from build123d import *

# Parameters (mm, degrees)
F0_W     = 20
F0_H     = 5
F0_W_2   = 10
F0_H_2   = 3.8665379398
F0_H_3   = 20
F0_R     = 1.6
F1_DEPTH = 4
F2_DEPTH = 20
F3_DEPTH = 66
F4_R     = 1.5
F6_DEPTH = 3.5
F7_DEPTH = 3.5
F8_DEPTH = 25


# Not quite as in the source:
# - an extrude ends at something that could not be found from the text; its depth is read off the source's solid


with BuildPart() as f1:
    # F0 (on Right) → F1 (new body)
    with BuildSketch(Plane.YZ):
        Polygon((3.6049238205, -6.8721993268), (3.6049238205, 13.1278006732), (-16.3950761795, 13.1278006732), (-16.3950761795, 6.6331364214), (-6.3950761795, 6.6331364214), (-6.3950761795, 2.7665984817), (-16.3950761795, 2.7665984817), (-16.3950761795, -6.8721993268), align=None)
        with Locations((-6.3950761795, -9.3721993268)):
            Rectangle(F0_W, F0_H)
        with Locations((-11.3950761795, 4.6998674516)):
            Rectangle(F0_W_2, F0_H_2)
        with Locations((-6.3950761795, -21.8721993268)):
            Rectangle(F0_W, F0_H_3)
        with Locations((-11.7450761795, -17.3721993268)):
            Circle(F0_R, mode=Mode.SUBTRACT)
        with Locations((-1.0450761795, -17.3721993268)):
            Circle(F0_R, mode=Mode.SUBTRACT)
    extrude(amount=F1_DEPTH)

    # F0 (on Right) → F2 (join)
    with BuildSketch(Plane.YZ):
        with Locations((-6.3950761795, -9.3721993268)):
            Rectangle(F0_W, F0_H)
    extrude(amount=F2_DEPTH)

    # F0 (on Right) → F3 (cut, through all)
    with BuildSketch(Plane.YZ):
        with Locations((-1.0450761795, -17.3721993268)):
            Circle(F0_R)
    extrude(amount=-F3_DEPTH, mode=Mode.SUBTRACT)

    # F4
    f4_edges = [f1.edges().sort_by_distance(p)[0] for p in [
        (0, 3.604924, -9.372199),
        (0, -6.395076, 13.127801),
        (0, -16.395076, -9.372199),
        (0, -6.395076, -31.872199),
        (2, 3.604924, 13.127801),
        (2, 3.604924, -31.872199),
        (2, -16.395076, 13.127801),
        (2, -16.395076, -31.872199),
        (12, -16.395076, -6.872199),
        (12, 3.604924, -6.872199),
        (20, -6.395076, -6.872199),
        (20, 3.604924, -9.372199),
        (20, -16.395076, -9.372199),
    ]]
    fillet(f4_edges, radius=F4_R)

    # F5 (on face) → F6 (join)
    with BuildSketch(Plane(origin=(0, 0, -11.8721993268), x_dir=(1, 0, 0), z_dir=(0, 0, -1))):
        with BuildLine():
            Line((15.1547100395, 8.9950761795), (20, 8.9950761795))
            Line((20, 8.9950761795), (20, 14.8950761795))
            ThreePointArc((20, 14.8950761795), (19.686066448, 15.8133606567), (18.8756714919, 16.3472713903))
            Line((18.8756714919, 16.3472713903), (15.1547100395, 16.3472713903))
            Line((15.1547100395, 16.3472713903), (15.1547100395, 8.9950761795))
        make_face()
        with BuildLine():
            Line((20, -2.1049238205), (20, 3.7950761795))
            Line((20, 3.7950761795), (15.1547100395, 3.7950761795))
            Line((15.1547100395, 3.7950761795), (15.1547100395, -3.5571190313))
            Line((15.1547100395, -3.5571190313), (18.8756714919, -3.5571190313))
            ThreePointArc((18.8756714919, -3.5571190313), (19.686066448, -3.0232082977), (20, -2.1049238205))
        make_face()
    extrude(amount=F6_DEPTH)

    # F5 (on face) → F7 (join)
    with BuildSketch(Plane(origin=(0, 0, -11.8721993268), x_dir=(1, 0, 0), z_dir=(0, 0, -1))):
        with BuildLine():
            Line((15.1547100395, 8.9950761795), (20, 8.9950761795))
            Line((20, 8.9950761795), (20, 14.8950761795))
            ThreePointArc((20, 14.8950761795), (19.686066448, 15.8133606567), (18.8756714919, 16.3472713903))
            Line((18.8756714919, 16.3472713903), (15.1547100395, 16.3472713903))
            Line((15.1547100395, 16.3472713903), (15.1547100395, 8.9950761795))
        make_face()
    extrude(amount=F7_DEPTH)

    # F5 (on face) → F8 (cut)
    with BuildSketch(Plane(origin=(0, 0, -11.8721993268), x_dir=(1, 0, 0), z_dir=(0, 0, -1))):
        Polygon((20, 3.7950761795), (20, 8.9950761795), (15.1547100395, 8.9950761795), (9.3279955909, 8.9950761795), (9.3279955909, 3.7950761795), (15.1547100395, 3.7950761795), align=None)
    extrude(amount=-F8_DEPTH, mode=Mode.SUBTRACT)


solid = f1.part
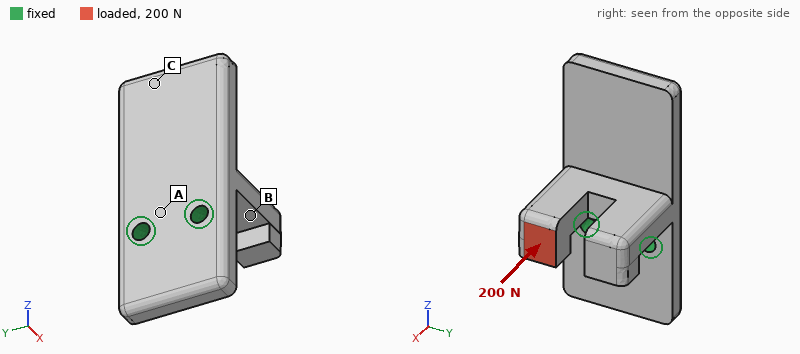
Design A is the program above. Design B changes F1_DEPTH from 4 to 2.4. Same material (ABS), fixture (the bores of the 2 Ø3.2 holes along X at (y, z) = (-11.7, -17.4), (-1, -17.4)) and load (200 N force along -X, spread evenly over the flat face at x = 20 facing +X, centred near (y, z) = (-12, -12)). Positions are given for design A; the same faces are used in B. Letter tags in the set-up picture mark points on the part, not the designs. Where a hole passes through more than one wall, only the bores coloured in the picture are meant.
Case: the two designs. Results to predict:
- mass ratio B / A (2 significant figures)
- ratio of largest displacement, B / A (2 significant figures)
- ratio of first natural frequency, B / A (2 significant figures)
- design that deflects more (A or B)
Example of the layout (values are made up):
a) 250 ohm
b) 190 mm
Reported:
a) 0.75
b) 3.7
c) 0.59
d) B
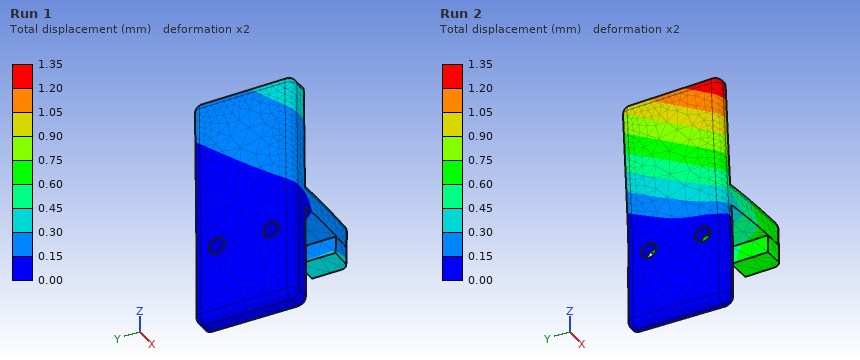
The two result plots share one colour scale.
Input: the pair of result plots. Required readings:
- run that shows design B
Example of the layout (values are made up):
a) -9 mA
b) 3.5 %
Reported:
a) Run 2
